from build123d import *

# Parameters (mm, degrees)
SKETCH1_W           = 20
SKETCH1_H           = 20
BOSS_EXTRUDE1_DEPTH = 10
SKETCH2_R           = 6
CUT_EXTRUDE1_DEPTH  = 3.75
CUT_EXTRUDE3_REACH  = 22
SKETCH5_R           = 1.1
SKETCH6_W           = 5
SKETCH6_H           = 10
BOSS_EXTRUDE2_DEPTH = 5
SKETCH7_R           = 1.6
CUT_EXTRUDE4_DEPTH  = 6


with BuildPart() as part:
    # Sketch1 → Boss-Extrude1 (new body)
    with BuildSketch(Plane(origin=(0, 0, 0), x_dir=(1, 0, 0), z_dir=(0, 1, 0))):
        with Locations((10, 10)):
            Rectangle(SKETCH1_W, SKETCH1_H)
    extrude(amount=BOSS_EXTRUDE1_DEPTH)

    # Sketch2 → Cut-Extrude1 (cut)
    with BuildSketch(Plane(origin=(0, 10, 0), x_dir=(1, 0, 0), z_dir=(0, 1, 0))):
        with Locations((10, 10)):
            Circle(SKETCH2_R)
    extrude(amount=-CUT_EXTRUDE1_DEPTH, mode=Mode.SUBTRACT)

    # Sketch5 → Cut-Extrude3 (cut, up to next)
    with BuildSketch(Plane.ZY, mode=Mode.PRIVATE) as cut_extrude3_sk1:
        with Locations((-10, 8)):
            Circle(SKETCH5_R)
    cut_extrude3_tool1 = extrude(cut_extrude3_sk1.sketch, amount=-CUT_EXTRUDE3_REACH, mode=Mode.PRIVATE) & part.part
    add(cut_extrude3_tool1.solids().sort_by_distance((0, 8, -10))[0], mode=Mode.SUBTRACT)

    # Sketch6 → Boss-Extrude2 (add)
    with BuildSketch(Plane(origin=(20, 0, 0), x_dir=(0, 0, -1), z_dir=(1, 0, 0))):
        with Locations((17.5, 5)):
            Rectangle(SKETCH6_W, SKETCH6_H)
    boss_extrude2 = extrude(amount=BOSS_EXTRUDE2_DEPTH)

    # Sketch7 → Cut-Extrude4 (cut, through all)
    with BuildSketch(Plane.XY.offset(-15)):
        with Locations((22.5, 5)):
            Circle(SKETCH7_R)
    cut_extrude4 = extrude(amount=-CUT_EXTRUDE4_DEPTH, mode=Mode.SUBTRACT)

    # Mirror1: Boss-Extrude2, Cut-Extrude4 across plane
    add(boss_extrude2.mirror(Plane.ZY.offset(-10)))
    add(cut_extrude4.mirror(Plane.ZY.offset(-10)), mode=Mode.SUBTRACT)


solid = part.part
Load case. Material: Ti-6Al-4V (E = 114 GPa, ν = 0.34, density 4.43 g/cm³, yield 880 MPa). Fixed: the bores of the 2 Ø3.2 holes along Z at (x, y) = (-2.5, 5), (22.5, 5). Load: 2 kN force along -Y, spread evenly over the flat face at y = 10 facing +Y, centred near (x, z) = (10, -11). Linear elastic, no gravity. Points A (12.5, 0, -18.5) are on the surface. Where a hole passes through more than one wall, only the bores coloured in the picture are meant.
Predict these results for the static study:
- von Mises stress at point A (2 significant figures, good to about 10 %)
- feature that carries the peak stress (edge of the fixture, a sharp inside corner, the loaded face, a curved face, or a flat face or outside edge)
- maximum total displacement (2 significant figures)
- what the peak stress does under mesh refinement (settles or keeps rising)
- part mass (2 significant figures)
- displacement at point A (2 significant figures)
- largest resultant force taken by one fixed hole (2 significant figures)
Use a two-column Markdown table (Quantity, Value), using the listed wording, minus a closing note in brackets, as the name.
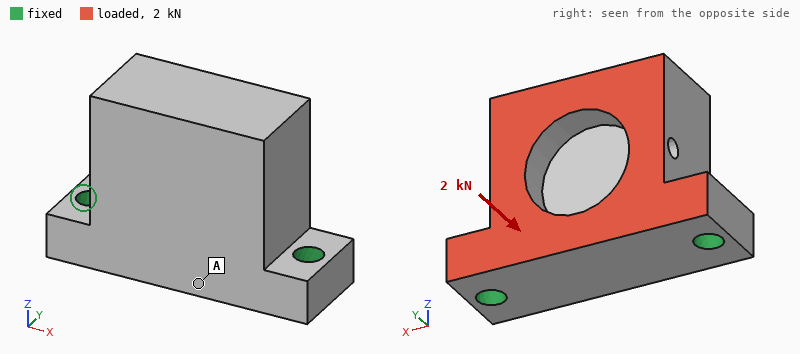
| Quantity | Value |
|---|---|
| von Mises stress at point A | 26 MPa |
| feature that carries the peak stress | edge of the fixture |
| maximum total displacement | 44 µm |
| what the peak stress does under mesh refinement | keeps rising |
| part mass | 18 g |
| displacement at point A | 9.5 µm |
| largest resultant force taken by one fixed hole | 1.0 kN |
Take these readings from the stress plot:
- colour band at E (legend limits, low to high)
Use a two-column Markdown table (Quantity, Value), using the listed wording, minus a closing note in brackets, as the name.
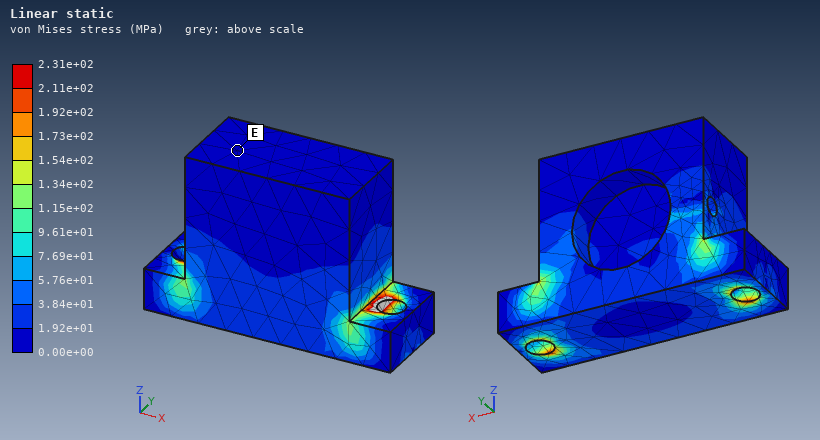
| Quantity | Value |
|---|---|
| colour band at E | 0.00e+00 to 1.92e+01 MPa |
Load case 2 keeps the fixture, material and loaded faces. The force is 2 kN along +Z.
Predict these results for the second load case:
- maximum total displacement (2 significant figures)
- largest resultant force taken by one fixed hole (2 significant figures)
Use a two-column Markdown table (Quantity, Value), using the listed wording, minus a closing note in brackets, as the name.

| Quantity | Value |
|---|---|
| maximum total displacement | 30 µm |
| largest resultant force taken by one fixed hole | 1.0 kN |
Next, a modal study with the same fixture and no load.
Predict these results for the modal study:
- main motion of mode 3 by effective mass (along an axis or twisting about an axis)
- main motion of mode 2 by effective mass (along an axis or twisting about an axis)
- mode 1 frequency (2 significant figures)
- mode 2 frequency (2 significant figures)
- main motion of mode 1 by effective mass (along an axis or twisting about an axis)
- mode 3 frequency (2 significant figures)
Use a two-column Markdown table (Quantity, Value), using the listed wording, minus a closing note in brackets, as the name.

| Quantity | Value |
|---|---|
| main motion of mode 3 by effective mass | along X |
| main motion of mode 2 by effective mass | along X |
| mode 1 frequency | 9500 Hz |
| mode 2 frequency | 23 kHz |
| main motion of mode 1 by effective mass | along Y |
| mode 3 frequency | 28 kHz |
